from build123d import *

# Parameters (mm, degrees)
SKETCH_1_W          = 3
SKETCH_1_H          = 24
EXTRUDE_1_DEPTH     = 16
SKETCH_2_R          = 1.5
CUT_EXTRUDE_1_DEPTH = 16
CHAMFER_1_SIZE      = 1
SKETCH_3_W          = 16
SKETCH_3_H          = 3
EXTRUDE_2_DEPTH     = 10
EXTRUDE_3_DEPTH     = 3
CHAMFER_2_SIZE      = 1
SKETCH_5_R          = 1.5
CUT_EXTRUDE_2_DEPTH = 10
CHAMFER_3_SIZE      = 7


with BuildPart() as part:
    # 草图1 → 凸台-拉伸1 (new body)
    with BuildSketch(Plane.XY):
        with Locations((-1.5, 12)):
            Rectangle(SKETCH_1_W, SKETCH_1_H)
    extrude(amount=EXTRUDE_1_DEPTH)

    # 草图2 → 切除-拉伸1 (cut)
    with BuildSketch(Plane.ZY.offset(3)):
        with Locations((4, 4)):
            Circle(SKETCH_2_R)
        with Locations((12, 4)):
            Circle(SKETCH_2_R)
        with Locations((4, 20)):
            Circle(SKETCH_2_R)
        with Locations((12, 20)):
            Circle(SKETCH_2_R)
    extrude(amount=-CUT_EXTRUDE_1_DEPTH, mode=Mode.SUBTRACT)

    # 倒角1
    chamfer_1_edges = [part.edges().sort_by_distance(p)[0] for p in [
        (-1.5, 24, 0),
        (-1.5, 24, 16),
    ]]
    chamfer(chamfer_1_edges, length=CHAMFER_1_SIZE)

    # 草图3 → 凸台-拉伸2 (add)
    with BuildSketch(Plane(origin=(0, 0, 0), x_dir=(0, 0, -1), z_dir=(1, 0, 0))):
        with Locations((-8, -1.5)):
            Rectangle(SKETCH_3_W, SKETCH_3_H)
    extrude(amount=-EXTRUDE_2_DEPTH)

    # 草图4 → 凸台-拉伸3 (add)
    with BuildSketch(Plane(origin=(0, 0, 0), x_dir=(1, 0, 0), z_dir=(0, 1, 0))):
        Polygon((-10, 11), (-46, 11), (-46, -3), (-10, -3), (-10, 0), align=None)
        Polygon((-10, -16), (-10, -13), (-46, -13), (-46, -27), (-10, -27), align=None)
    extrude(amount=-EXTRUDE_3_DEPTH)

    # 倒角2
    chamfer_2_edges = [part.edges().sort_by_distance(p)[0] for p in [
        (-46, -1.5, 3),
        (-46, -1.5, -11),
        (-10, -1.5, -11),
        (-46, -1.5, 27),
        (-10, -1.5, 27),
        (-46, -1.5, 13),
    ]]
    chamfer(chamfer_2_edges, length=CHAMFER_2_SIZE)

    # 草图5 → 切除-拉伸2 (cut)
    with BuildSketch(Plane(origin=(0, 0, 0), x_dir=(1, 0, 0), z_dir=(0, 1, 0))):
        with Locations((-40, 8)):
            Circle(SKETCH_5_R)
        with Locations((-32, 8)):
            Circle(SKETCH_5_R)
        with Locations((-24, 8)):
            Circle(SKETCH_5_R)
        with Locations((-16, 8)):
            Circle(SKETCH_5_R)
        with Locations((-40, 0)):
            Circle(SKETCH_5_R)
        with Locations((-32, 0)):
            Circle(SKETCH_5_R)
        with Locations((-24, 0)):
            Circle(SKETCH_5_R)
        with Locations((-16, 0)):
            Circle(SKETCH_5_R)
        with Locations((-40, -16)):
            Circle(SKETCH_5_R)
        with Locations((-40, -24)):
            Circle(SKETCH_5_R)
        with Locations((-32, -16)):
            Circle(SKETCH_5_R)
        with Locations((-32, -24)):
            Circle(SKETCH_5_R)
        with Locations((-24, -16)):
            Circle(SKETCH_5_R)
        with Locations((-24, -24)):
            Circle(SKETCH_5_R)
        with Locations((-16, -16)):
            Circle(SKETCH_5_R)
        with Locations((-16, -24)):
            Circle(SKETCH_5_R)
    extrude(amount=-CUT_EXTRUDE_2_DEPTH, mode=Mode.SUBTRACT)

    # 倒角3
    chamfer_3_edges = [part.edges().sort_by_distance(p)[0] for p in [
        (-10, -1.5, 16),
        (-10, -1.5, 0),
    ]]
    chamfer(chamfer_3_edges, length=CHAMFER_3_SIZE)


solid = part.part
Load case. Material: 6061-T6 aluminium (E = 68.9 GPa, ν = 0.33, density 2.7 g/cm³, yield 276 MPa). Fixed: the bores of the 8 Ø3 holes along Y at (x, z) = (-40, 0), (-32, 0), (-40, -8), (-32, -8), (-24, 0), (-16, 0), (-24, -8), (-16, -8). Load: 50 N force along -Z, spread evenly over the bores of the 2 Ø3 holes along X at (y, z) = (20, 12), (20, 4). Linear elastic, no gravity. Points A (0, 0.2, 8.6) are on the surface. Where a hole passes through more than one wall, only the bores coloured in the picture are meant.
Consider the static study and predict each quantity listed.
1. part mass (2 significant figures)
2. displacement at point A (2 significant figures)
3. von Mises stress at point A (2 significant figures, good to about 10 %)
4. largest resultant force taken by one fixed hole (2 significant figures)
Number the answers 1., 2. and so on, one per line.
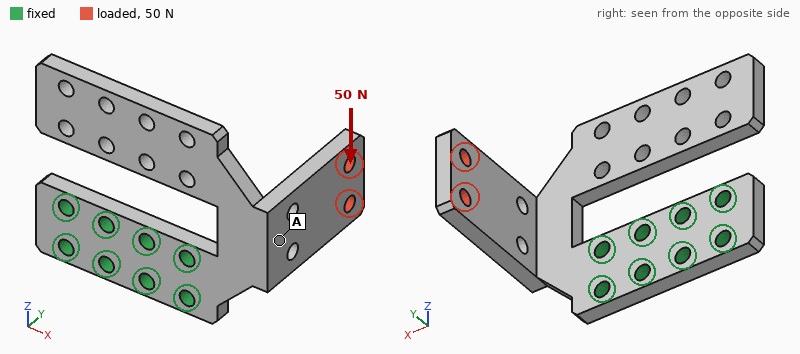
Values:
1. 12 g
2. 0.070 mm
3. 15 MPa
4. 130 N
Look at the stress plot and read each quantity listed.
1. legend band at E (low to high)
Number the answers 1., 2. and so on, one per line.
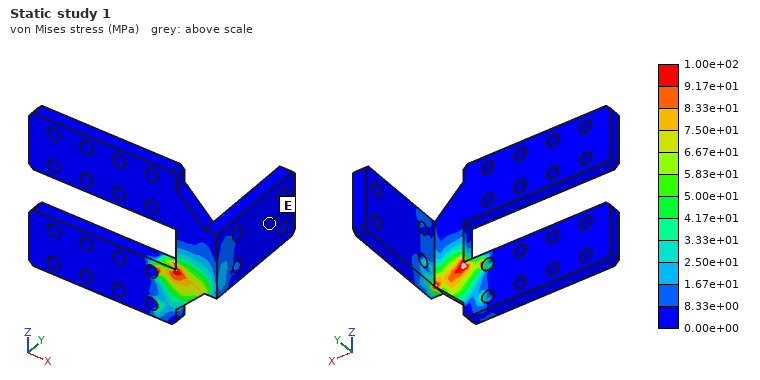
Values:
1. 0.00e+00 to 8.33e+00 MPa
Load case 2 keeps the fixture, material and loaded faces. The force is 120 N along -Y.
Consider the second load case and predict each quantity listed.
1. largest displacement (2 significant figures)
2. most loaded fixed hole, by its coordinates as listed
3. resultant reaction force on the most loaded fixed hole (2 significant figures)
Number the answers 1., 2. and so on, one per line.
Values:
1. 0.34 mm
2. (-16, 0)
3. 210 N
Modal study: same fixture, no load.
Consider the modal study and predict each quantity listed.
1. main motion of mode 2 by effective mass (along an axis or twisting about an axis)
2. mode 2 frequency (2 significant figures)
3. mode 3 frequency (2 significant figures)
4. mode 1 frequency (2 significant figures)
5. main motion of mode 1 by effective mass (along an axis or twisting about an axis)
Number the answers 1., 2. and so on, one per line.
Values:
1. along Y
2. 1400 Hz
3. 1800 Hz
4. 730 Hz
5. along Y
